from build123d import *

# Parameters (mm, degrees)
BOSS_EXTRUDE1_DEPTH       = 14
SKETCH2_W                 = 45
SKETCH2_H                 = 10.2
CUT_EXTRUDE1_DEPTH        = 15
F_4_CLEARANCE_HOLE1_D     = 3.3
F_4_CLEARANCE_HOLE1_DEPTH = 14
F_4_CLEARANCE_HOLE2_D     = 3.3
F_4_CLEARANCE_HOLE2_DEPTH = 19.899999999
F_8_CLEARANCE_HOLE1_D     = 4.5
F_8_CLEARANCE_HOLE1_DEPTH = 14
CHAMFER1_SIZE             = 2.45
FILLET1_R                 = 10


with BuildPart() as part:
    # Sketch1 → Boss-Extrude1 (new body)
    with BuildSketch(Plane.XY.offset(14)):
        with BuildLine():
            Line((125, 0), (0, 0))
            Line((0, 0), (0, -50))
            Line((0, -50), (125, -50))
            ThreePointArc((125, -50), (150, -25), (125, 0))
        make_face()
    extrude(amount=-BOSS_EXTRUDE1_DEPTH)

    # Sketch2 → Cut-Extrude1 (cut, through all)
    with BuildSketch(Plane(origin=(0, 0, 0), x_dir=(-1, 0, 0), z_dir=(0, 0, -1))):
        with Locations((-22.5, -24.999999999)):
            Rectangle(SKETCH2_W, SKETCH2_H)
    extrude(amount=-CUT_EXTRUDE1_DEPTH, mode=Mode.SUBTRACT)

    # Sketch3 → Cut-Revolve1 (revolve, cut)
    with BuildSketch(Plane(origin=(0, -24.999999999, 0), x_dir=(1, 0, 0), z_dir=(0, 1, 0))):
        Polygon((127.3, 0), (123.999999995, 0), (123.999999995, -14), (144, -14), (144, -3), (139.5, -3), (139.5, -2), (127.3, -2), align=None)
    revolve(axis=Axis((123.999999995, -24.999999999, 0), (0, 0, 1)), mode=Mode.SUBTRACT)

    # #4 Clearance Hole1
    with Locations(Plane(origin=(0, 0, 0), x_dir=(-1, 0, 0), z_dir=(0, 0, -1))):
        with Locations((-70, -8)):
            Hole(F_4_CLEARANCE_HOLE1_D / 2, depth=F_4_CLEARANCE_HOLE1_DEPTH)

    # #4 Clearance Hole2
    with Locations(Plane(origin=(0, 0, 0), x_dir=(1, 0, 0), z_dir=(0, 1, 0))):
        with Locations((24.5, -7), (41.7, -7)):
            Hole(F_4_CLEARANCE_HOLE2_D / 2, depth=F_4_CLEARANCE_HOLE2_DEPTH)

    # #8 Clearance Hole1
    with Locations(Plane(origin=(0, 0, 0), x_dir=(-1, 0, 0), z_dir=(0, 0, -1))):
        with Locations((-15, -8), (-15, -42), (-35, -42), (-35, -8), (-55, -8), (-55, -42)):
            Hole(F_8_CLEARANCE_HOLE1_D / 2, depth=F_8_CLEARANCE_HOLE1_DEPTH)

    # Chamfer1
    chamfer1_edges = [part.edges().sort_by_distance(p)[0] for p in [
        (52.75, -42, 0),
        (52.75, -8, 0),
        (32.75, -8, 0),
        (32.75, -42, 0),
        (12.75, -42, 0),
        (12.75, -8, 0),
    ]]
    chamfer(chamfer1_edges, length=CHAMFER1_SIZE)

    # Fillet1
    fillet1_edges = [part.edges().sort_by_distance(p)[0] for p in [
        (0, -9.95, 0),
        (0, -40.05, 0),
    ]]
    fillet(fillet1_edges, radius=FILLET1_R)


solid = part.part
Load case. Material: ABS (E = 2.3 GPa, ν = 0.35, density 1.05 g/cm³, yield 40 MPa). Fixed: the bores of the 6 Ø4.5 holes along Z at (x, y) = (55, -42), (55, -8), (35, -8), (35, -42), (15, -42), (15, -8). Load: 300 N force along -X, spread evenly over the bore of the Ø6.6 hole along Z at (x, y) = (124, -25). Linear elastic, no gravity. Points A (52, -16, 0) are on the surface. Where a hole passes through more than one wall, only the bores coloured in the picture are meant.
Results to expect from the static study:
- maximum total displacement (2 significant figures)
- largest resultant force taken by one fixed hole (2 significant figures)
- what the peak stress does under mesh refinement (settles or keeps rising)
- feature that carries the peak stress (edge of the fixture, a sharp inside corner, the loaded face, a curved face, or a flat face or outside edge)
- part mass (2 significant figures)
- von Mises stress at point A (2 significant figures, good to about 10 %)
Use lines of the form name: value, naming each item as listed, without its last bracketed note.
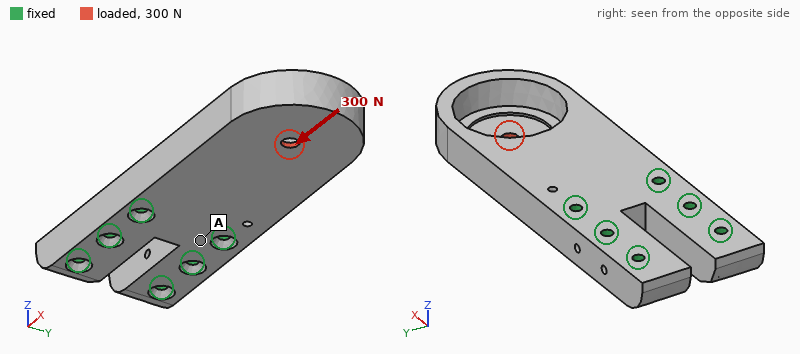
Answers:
maximum total displacement: 0.33 mm
largest resultant force taken by one fixed hole: 120 N
what the peak stress does under mesh refinement: keeps rising
feature that carries the peak stress: a sharp inside corner
part mass: 81 g
von Mises stress at point A: 0.97 MPa
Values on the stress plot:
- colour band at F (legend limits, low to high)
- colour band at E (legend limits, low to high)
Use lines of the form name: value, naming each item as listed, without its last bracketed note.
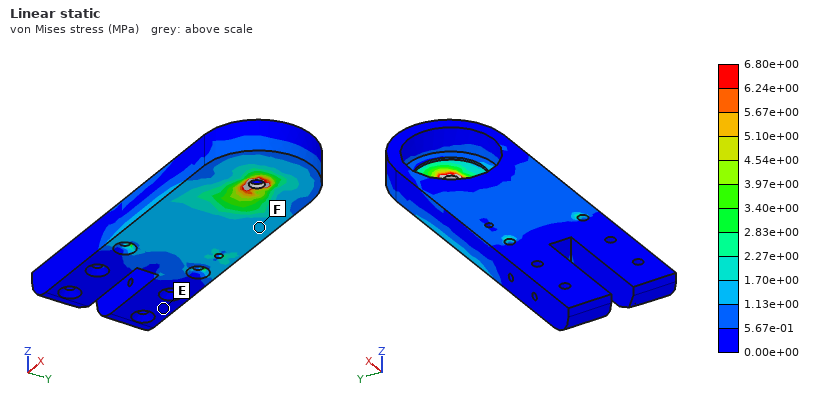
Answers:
colour band at F: 1.13e+00 to 1.70e+00 MPa
colour band at E: 0.00e+00 to 5.67e-01 MPa
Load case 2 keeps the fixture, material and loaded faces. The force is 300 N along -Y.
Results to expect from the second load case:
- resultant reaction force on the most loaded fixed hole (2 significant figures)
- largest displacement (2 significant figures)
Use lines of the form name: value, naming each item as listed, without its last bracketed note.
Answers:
resultant reaction force on the most loaded fixed hole: 520 N
largest displacement: 0.28 mm
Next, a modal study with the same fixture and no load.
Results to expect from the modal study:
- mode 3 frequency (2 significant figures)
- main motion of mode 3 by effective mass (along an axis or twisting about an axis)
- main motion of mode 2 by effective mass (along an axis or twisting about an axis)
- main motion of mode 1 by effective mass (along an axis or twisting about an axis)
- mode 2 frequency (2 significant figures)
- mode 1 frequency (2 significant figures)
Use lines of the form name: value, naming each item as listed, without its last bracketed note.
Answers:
mode 3 frequency: 1500 Hz
main motion of mode 3 by effective mass: along Y
main motion of mode 2 by effective mass: along Y
main motion of mode 1 by effective mass: along Z
mode 2 frequency: 1300 Hz
mode 1 frequency: 480 Hz
